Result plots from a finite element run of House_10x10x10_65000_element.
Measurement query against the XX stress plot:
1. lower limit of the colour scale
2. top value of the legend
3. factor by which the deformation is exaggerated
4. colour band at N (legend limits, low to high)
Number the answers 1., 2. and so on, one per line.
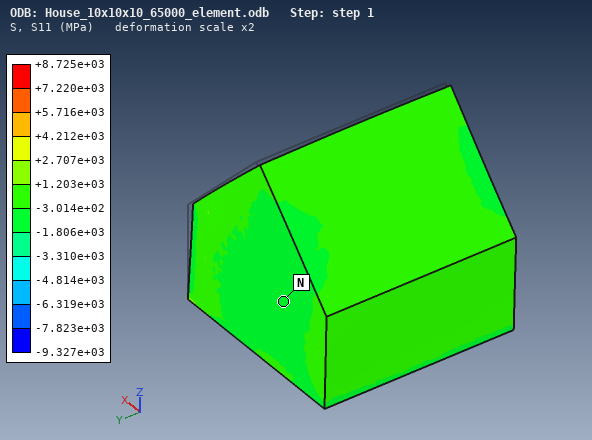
1. -9.327e+03 MPa
2. +8.725e+03 MPa
3. 2
4. -1.806e+03 to -3.014e+02 MPa
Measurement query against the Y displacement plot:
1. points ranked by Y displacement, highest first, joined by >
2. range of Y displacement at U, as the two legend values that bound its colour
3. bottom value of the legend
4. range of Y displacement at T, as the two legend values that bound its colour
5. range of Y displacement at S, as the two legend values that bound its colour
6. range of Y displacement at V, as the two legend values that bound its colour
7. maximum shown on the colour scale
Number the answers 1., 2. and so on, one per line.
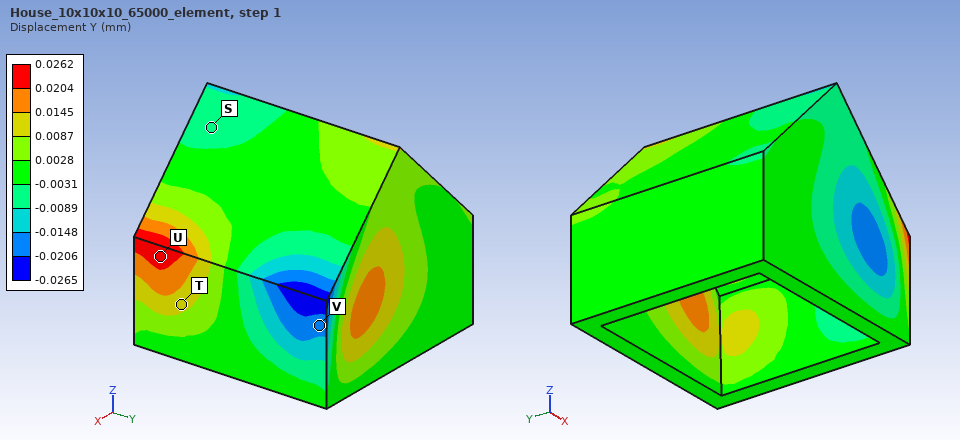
1. U > T > S > V
2. 0.0204 to 0.0262 mm
3. -0.0265 mm
4. 0.0087 to 0.0145 mm
5. -0.0089 to -0.0031 mm
6. -0.0206 to -0.0148 mm
7. 0.0262 mm
